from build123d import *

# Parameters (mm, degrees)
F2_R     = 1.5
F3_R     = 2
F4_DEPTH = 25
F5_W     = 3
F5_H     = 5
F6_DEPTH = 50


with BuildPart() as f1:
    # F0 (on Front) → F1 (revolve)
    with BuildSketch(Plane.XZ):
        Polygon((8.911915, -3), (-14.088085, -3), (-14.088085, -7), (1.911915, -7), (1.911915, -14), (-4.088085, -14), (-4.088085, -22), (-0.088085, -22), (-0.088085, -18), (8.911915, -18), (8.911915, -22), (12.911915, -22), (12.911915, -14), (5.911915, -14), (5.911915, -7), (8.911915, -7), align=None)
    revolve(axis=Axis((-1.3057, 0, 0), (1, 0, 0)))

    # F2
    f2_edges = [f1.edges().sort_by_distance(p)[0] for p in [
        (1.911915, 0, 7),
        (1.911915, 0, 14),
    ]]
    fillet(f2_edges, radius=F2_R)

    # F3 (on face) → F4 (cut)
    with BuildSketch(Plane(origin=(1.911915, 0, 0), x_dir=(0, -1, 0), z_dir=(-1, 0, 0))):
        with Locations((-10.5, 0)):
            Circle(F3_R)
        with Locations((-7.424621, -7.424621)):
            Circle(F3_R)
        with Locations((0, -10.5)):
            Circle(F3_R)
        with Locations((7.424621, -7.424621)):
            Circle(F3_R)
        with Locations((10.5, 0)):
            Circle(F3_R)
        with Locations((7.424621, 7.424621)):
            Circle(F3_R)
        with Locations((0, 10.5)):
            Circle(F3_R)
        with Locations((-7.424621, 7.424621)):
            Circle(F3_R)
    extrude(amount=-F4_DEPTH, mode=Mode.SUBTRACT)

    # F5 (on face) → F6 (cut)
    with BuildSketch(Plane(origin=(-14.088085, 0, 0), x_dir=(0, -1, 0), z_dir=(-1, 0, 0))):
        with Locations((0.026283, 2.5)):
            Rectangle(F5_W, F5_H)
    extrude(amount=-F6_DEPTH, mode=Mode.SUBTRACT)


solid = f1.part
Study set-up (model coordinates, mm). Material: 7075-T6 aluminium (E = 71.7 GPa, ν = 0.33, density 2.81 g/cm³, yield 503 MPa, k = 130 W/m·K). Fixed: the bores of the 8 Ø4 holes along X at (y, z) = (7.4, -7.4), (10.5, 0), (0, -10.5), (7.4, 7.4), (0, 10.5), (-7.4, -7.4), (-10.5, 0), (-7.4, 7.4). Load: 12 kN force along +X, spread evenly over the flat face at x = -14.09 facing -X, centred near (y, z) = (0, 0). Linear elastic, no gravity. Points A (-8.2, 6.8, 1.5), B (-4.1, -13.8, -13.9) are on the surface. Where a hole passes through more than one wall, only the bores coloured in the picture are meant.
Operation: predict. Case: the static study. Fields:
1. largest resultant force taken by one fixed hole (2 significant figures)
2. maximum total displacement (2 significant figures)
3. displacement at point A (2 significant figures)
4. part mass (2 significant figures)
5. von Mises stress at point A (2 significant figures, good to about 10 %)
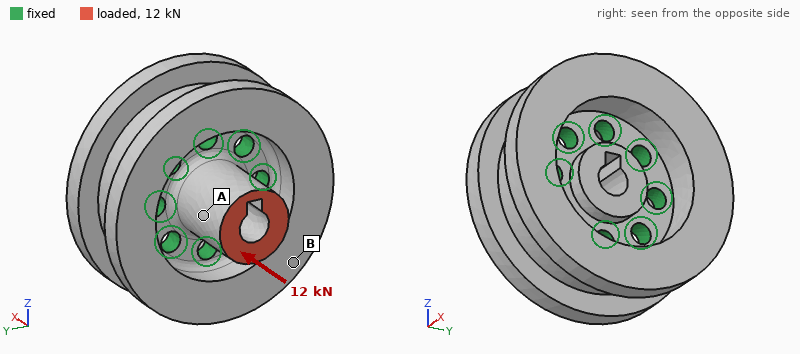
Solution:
1.7 kN
31 µm
22 µm
42 g
96 MPa
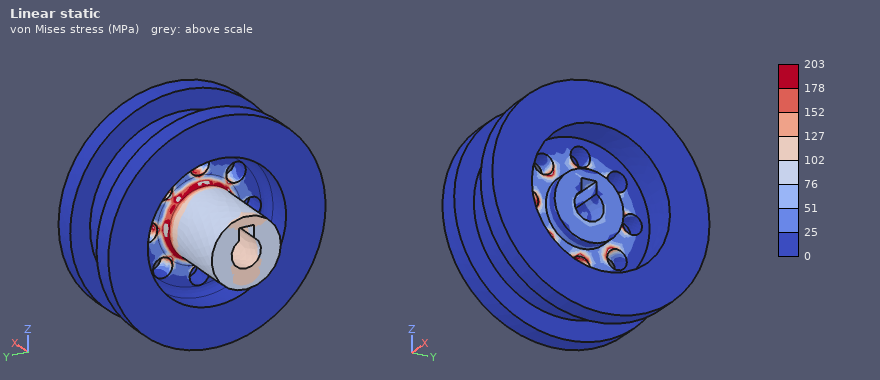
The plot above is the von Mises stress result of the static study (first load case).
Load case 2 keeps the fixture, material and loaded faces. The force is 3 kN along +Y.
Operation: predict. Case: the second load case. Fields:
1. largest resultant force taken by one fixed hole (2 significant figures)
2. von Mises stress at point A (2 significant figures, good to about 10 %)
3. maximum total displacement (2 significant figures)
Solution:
1.7 kN
79 MPa
85 µm
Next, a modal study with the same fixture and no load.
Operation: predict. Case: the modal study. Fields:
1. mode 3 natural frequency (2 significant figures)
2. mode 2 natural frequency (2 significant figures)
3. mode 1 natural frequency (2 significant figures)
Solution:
21 kHz
20 kHz
20 kHz
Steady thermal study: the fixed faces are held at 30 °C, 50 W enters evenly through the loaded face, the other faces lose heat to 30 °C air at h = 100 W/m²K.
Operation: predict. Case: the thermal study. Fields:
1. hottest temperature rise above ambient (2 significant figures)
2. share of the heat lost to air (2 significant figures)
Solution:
57 K
7.3 %
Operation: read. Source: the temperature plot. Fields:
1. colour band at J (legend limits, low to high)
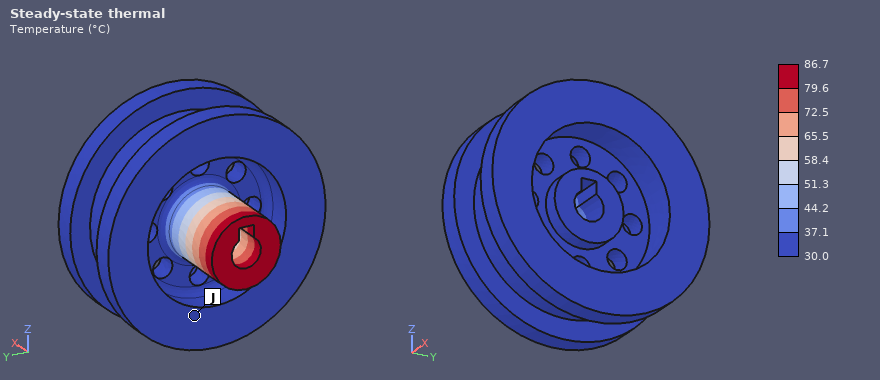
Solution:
30.0 to 37.1 °C
